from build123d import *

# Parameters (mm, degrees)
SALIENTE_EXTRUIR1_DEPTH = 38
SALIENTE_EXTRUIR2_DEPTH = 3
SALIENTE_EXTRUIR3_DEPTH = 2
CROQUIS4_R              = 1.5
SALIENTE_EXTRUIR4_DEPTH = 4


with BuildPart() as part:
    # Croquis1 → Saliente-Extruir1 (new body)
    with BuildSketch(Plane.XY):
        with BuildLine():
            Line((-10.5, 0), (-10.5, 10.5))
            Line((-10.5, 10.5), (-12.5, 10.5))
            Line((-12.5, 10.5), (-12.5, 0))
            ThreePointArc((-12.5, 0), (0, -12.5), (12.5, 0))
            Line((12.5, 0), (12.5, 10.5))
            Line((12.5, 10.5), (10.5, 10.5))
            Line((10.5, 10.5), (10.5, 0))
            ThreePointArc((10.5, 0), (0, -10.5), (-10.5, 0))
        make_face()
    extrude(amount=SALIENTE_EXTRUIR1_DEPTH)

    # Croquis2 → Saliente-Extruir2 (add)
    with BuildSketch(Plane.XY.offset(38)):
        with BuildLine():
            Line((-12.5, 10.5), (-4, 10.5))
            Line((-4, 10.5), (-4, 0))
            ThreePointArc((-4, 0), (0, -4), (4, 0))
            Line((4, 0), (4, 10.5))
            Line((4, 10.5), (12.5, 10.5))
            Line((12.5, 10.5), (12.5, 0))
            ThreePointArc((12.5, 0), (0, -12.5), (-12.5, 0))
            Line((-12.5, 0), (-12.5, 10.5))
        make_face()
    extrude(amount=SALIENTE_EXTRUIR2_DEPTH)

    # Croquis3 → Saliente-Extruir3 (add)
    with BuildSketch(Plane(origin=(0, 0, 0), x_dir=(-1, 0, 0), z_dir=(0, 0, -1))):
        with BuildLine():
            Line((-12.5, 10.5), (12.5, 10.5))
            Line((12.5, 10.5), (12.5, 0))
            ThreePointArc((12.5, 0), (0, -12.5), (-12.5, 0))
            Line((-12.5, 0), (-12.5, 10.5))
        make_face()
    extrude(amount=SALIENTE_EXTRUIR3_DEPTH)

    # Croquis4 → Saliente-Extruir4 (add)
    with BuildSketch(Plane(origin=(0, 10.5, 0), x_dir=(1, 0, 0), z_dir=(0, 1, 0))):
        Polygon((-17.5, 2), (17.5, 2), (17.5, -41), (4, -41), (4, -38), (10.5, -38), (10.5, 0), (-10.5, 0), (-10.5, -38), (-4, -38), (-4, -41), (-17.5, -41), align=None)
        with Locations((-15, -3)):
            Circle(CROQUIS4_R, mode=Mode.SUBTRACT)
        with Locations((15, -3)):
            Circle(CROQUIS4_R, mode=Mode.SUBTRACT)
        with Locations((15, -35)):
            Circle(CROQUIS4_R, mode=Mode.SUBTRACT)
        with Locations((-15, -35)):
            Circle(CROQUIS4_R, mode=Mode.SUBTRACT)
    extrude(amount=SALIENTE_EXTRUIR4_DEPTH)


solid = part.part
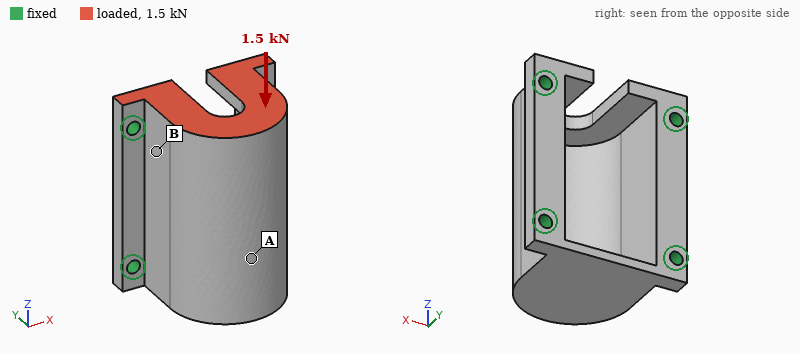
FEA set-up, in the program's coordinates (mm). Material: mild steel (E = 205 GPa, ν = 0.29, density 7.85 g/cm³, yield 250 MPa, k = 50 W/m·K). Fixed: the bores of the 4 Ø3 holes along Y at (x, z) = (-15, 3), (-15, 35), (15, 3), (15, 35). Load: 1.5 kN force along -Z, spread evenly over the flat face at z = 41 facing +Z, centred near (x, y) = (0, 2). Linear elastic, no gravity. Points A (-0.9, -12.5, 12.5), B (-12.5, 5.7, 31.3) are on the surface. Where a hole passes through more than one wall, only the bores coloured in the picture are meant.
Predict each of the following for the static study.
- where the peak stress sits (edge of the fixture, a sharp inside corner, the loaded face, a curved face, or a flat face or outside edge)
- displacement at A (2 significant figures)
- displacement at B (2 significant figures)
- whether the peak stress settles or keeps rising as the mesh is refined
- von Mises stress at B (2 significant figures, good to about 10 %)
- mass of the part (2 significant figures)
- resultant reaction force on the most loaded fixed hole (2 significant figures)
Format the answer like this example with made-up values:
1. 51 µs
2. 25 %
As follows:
1. edge of the fixture
2. 2.7 µm
3. 1.9 µm
4. keeps rising
5. 21 MPa
6. 72 g
7. 530 N
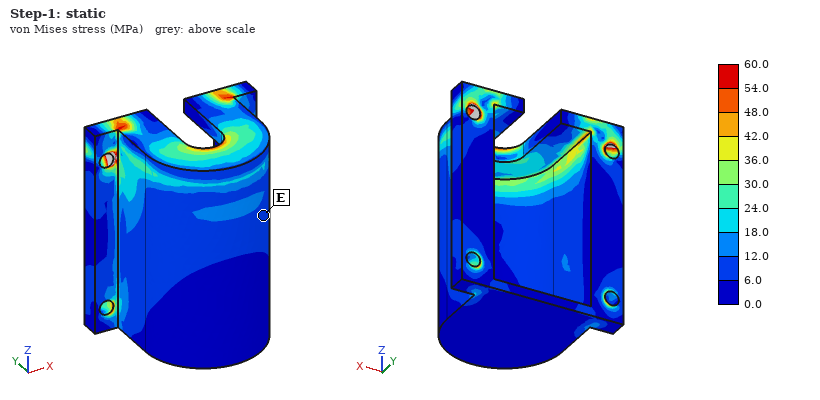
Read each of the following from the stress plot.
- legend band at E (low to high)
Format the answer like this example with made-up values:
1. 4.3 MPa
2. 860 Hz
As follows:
1. 6.0 to 12.0 MPa
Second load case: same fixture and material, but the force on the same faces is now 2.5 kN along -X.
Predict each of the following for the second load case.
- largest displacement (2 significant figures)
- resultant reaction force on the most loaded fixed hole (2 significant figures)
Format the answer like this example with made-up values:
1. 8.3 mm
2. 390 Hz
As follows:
1. 23 µm
2. 1.3 kN
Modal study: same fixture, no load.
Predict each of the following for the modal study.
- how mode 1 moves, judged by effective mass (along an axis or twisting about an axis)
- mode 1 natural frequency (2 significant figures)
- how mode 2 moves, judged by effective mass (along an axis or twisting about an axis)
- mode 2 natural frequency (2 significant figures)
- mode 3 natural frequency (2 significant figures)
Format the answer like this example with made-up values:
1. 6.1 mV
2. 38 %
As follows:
1. along X
2. 9700 Hz
3. along Z
4. 14 kHz
5. 15 kHz
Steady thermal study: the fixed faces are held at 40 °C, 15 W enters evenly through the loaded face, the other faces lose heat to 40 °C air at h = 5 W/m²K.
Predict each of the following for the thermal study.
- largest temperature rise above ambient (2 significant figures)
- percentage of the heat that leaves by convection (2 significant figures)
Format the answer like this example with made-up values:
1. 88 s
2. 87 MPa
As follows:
1. 37 K
2. 3.2 %
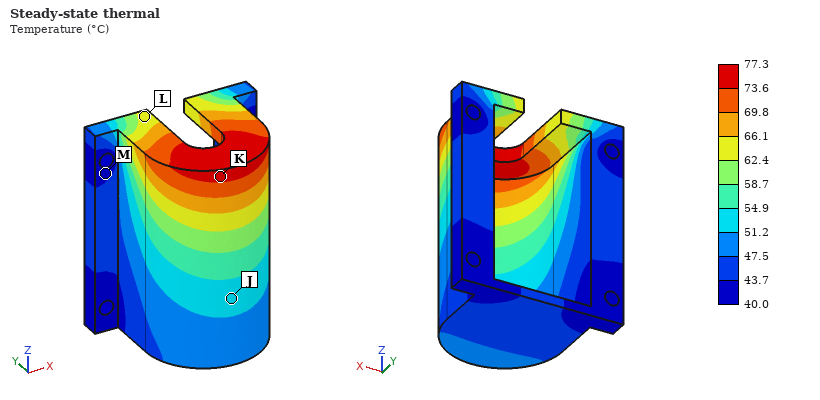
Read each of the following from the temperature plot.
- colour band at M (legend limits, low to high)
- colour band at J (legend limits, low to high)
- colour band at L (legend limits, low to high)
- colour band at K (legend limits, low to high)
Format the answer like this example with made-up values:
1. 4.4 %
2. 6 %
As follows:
1. 40.0 to 43.7 °C
2. 51.2 to 54.9 °C
3. 62.4 to 66.1 °C
4. 73.6 to 77.3 °C
